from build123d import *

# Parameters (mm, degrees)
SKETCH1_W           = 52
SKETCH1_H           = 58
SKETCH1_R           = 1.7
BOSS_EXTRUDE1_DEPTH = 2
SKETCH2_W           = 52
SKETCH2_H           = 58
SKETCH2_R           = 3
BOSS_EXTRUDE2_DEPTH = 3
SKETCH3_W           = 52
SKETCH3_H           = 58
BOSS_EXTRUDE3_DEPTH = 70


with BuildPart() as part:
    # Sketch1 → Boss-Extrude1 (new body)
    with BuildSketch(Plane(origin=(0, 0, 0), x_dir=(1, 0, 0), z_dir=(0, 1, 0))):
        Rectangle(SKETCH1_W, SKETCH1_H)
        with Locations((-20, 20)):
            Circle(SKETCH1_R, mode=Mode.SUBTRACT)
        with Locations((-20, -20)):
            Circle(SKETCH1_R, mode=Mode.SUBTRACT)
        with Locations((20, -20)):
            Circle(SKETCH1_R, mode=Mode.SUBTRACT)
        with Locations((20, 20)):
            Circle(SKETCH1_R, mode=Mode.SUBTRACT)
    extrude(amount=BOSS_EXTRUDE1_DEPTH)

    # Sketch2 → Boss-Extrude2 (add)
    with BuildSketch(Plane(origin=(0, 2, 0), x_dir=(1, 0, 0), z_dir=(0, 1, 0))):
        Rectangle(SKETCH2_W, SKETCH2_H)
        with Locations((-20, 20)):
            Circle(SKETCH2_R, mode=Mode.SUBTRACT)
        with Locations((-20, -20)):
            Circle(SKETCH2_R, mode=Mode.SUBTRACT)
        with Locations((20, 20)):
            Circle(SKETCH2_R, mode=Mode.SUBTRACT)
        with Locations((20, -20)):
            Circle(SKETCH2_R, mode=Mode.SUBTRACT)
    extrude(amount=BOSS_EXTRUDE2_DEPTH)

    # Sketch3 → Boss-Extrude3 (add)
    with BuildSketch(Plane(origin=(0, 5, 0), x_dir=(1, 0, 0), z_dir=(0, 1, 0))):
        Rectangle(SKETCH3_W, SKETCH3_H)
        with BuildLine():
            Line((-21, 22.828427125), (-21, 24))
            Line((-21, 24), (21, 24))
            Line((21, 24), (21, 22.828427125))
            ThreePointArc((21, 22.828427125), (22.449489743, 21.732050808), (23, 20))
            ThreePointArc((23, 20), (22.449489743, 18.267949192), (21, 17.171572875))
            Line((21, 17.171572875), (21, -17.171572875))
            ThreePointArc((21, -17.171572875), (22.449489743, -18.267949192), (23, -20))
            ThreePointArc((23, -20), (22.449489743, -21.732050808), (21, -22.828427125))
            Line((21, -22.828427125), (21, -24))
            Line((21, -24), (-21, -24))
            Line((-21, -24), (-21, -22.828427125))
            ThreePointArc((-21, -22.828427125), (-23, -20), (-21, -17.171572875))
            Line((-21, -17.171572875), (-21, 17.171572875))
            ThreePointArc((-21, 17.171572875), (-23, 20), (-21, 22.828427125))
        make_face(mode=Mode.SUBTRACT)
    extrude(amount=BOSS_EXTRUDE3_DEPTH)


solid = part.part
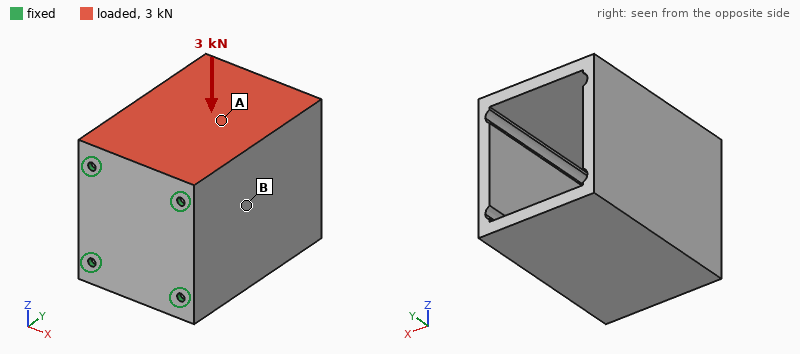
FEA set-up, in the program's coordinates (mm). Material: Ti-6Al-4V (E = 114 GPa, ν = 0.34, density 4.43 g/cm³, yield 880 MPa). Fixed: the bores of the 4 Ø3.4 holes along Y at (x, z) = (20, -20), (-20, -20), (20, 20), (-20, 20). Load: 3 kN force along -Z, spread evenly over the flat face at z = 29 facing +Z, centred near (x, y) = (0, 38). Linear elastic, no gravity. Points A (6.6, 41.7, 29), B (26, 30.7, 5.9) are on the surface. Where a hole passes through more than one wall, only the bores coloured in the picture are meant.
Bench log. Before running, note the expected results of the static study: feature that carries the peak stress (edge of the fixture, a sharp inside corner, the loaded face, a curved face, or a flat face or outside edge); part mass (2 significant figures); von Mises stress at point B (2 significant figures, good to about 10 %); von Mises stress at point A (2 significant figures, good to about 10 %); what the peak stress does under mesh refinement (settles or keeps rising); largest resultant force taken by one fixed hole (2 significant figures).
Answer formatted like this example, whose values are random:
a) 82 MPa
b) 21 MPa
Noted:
a) edge of the fixture
b) 360 g
c) 9.3 MPa
d) 23 MPa
e) keeps rising
f) 1.5 kN
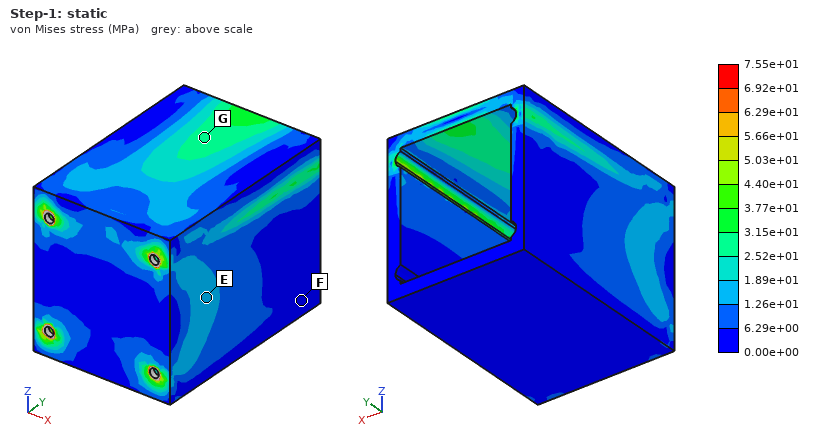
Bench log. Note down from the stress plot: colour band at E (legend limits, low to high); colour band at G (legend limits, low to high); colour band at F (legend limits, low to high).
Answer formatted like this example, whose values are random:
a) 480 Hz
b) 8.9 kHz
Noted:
a) 1.26e+01 to 1.89e+01 MPa
b) 2.52e+01 to 3.15e+01 MPa
c) 0.00e+00 to 6.29e+00 MPa
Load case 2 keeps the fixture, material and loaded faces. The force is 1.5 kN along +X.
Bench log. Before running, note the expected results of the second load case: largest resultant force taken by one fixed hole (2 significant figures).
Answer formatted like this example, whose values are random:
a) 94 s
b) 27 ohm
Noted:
a) 1.3 kN
